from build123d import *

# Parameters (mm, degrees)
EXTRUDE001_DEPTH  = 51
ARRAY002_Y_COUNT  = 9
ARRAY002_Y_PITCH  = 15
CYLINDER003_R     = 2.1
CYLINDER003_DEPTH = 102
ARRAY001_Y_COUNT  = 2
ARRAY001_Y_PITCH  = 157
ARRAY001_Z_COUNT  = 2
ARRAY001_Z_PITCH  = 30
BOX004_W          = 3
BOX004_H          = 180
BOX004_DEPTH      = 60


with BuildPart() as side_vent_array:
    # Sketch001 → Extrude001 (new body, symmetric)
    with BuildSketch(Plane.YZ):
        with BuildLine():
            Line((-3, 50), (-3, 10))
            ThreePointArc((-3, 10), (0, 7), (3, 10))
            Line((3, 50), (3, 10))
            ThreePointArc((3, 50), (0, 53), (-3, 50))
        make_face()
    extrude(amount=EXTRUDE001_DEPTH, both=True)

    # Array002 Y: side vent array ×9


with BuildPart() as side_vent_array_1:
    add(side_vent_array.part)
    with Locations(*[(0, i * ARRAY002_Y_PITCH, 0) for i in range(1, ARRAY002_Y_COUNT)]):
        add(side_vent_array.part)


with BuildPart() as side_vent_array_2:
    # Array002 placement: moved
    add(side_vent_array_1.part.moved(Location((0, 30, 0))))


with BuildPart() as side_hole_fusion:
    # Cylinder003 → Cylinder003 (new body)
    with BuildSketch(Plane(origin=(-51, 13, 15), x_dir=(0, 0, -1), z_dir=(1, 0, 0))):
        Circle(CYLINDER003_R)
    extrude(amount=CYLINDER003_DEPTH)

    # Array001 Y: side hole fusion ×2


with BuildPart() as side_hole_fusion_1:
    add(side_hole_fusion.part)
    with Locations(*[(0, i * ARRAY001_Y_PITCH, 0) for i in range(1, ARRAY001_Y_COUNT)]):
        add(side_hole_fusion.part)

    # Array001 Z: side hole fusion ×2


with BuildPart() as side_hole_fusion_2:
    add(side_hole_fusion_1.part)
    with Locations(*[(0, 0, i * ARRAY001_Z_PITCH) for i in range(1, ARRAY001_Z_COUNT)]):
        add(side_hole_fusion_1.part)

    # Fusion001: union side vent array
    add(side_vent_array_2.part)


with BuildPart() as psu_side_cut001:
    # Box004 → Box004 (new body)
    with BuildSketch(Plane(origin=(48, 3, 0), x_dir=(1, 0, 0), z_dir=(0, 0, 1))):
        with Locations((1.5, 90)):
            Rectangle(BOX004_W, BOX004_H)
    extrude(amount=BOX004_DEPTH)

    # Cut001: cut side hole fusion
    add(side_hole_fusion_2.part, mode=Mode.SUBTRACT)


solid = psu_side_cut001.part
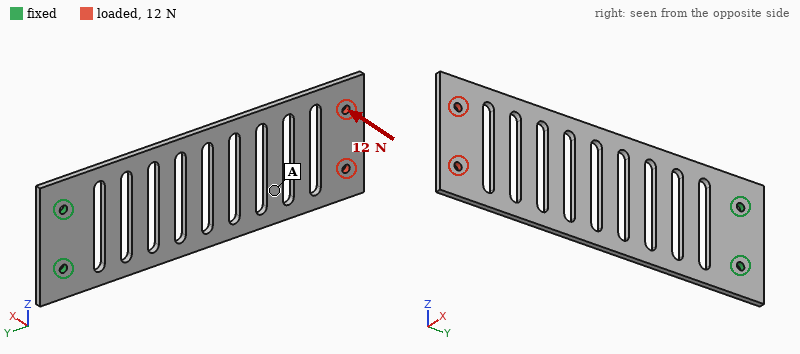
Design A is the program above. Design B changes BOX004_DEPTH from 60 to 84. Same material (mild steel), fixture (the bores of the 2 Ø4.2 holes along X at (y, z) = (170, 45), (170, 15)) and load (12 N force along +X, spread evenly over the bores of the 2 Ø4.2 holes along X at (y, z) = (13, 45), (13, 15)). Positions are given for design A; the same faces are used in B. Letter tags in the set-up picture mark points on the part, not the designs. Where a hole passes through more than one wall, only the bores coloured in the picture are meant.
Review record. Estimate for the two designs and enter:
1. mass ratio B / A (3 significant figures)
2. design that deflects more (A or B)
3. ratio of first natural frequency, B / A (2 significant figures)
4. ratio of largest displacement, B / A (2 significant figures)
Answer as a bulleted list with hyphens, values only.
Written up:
- 1.52
- A
- 1.2
- 0.50
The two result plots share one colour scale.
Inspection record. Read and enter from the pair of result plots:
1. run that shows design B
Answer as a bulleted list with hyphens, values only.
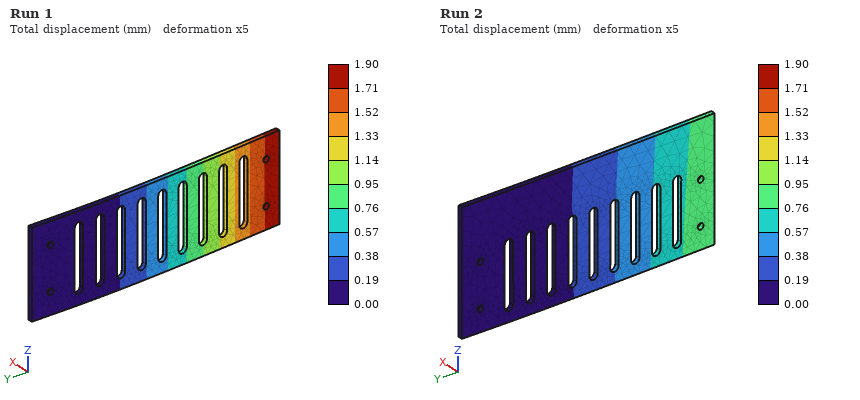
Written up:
- Run 2
